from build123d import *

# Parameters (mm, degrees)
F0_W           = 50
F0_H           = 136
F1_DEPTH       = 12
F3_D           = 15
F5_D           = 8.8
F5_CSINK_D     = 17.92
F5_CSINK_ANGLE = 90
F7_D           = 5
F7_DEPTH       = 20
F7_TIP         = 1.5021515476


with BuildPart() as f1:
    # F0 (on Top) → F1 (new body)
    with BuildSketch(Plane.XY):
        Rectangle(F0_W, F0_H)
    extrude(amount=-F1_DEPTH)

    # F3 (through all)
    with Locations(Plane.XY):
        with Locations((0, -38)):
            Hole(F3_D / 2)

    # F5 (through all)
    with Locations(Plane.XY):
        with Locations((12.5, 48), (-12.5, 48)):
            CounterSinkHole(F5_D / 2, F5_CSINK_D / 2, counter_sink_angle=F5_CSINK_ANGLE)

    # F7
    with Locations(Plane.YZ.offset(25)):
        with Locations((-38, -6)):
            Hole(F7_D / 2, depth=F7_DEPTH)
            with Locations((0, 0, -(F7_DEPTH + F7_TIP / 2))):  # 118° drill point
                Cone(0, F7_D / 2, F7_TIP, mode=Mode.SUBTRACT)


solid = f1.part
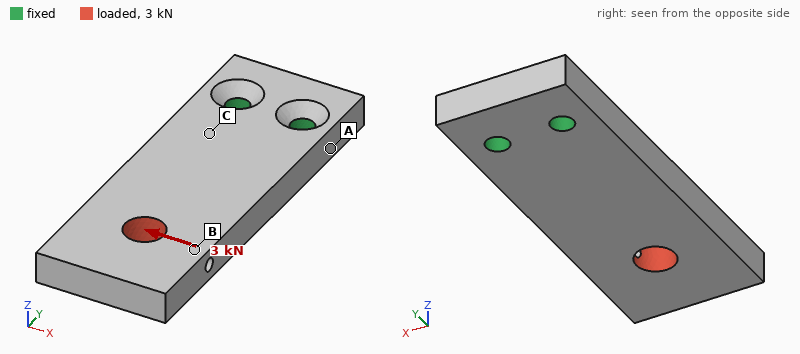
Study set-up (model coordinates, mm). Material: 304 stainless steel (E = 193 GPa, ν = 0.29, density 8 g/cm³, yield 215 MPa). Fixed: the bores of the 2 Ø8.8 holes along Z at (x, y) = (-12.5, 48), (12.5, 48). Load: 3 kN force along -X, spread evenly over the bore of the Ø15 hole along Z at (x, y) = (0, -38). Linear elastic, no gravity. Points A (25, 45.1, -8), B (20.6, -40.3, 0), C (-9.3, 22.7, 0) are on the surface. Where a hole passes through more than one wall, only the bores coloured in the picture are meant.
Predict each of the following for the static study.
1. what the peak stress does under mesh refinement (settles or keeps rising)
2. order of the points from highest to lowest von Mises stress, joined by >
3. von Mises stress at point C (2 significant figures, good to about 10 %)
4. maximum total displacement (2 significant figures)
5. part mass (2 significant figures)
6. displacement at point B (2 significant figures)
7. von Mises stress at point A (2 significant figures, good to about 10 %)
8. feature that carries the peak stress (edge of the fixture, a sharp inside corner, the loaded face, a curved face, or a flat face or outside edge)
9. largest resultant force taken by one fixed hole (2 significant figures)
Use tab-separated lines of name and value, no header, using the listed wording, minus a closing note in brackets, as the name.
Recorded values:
what the peak stress does under mesh refinement	keeps rising
order of the points from highest to lowest von Mises stress, joined by >	A > C > B
von Mises stress at point C	16 MPa
maximum total displacement	59 µm
part mass	620 g
displacement at point B	42 µm
von Mises stress at point A	33 MPa
feature that carries the peak stress	edge of the fixture
largest resultant force taken by one fixed hole	8.6 kN
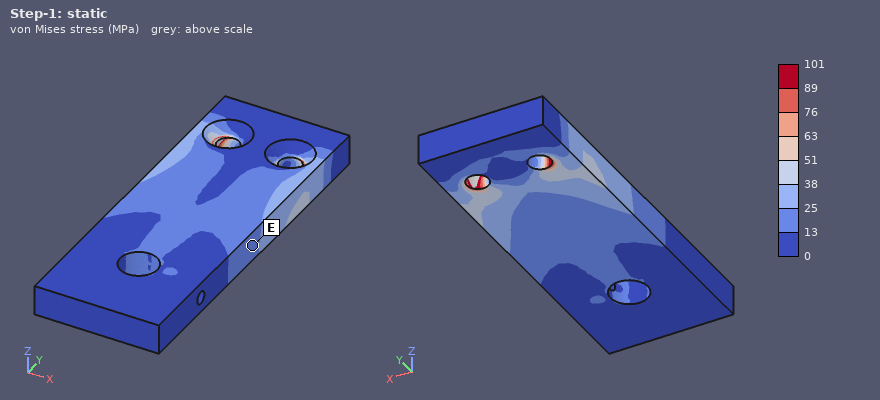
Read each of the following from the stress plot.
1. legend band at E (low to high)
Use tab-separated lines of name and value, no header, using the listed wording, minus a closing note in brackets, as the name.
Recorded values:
legend band at E	13 to 25 MPa
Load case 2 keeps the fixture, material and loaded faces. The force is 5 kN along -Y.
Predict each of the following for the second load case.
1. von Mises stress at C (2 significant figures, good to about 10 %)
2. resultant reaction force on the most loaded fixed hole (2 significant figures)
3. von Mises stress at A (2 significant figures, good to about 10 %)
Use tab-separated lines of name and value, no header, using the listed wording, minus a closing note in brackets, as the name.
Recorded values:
von Mises stress at C	8.7 MPa
resultant reaction force on the most loaded fixed hole	2.6 kN
von Mises stress at A	4.0 MPa
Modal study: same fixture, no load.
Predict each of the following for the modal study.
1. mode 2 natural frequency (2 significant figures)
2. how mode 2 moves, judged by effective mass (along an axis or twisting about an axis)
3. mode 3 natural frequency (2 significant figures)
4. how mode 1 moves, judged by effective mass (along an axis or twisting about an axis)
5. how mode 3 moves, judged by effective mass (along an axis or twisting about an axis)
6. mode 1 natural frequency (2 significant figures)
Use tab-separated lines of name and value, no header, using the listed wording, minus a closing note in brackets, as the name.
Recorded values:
mode 2 natural frequency	2400 Hz
how mode 2 moves, judged by effective mass	along X
mode 3 natural frequency	3000 Hz
how mode 1 moves, judged by effective mass	along Z
how mode 3 moves, judged by effective mass	twisting about Y
mode 1 natural frequency	670 Hz
